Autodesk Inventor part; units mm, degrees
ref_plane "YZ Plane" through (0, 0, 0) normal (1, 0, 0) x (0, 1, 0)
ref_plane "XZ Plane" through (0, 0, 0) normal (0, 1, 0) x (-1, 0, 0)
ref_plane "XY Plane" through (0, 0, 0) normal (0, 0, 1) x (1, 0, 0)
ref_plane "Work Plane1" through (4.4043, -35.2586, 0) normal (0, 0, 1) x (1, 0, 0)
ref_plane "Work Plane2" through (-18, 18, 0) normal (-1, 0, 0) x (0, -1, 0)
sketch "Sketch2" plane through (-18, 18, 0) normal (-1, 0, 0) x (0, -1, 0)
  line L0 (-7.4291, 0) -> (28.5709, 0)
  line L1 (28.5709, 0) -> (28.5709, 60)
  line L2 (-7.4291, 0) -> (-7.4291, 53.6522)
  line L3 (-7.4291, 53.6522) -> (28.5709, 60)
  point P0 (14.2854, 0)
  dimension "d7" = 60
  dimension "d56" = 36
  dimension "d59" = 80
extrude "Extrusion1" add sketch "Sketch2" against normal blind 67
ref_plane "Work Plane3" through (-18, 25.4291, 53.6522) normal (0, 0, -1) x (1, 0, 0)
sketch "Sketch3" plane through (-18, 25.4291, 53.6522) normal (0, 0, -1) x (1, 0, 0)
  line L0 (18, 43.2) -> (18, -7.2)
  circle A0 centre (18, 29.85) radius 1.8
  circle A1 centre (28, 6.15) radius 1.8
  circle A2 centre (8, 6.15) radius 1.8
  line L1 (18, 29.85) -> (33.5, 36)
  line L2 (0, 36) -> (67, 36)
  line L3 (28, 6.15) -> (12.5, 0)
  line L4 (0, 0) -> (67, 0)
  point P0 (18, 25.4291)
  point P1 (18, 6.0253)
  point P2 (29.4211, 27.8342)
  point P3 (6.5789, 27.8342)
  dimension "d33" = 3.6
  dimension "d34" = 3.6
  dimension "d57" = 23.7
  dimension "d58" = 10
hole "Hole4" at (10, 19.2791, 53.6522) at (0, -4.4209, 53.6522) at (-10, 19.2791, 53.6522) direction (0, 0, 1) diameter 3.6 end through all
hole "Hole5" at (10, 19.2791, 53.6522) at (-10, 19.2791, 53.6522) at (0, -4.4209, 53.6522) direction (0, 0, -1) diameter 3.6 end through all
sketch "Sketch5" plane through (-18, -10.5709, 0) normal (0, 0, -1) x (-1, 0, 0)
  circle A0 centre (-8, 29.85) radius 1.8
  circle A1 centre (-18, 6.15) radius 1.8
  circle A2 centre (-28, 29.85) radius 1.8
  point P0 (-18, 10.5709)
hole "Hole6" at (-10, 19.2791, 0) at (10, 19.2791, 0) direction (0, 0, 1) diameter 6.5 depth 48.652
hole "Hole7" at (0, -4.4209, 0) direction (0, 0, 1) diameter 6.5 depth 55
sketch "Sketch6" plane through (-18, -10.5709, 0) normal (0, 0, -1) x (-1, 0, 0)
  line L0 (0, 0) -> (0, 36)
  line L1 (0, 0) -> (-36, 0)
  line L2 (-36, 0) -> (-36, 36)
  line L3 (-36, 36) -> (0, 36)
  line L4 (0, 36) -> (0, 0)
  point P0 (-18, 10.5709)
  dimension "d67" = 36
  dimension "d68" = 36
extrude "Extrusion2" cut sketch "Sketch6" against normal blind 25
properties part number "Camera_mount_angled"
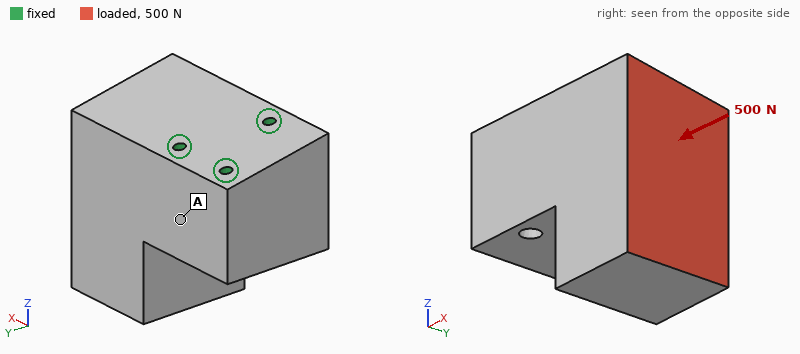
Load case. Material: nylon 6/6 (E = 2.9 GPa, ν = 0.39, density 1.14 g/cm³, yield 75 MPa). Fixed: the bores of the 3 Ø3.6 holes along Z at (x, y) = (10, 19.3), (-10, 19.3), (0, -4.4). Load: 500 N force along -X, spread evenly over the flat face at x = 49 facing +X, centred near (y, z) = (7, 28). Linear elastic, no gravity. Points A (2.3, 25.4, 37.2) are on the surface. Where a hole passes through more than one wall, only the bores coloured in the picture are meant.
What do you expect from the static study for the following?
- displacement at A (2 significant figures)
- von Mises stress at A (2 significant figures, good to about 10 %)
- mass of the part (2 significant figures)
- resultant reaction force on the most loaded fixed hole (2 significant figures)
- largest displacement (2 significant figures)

0.042 mm
2.4 MPa
120 g
580 N
0.26 mm
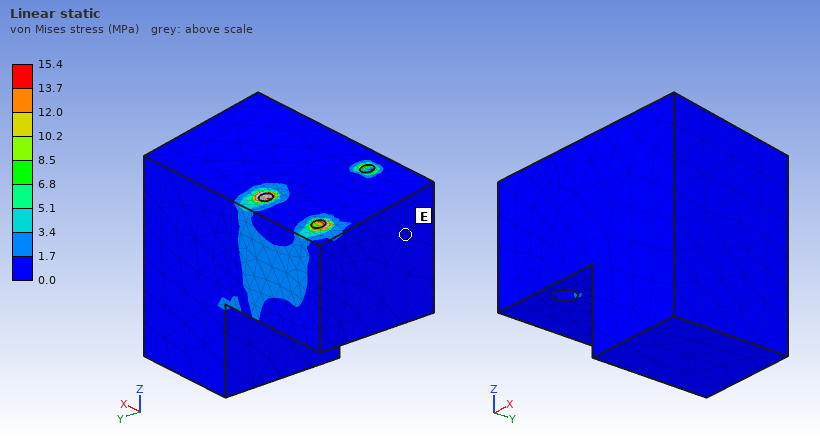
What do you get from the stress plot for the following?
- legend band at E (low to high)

0.0 to 1.7 MPa
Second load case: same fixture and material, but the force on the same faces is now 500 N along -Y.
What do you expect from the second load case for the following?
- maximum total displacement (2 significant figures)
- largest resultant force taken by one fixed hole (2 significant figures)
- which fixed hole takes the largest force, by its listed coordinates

0.27 mm
880 N
(10, 19.3)
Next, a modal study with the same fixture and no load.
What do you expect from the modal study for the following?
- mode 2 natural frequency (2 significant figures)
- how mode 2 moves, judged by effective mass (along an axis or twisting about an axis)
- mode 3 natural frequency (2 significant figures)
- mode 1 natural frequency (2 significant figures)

1100 Hz
along Y
2200 Hz
770 Hz
